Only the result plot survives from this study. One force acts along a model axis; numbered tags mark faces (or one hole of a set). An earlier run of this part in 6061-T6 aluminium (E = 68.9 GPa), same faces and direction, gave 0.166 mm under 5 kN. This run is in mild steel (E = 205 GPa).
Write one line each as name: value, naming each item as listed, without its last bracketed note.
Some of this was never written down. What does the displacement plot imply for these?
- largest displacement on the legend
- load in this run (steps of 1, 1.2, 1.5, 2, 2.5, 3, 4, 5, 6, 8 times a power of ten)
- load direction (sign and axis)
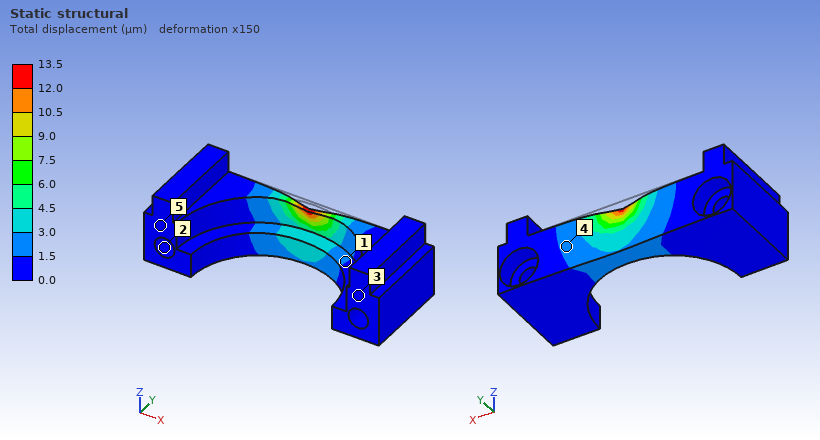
largest displacement on the legend: 13.5 µm
load in this run: 1.2 kN
load direction: -Y
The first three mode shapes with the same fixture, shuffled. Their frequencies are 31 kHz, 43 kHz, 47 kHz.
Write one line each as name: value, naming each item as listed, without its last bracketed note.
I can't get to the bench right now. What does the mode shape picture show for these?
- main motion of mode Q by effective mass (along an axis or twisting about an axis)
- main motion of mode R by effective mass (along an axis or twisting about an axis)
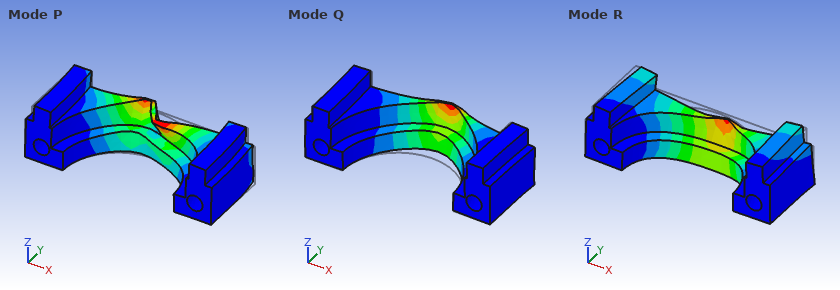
main motion of mode Q by effective mass: along Y
main motion of mode R by effective mass: along Z
